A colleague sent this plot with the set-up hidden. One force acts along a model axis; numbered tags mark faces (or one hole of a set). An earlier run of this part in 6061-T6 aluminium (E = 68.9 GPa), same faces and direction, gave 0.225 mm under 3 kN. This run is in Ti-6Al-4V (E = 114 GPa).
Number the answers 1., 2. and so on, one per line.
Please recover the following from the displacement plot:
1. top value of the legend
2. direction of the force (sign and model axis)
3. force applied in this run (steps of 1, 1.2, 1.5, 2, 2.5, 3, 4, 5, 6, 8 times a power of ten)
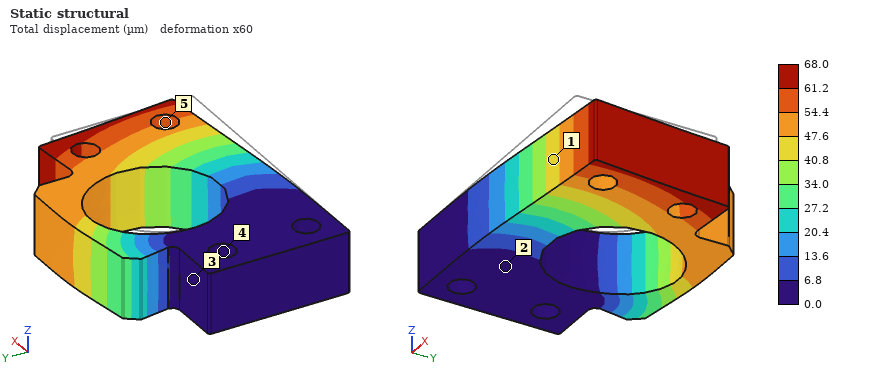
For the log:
1. 68.0 µm
2. +Y
3. 1.5 kN
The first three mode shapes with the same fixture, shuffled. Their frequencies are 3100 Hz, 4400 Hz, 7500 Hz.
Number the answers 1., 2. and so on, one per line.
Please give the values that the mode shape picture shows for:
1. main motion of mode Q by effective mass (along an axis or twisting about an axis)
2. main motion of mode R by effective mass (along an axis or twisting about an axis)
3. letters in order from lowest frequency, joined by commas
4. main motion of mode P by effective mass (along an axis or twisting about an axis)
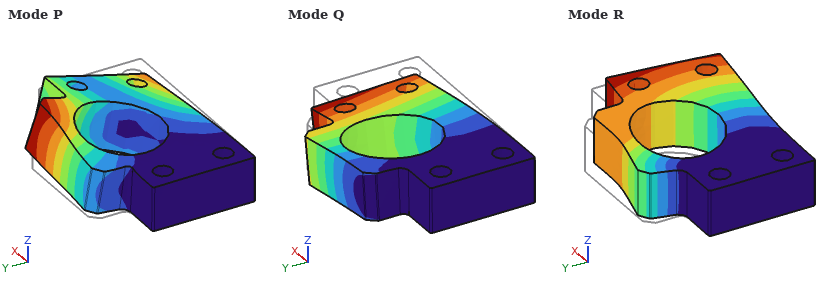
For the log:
1. along Z
2. along Y
3. Q, R, P
4. twisting about X
